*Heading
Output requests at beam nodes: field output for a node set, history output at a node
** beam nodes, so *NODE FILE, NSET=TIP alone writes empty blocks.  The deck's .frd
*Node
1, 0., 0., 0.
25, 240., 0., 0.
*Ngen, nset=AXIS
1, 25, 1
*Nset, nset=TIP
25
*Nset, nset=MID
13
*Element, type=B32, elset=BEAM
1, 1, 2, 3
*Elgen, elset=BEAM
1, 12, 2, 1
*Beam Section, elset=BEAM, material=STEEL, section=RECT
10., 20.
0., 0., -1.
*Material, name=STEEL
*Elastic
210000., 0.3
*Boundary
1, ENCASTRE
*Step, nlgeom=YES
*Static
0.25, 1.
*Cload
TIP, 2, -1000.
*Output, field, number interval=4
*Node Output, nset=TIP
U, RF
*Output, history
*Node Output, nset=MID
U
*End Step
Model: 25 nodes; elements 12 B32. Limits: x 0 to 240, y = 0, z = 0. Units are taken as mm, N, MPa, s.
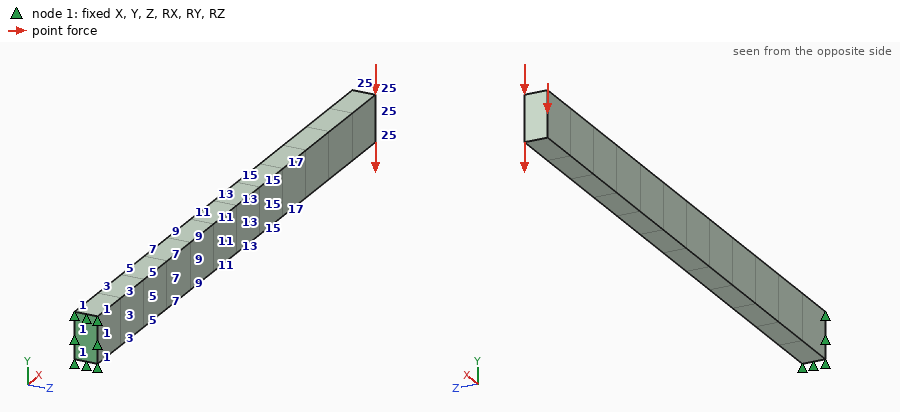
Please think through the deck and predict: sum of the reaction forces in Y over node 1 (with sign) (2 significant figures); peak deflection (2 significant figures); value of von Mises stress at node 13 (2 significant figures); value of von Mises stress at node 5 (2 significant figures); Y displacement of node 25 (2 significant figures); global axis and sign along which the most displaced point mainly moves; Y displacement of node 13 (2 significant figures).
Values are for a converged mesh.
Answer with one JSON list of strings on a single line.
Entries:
["1000 N", "3.3 mm", "180 MPa", "300 MPa", "-3.3 mm", "-Y", "-1.0 mm"]
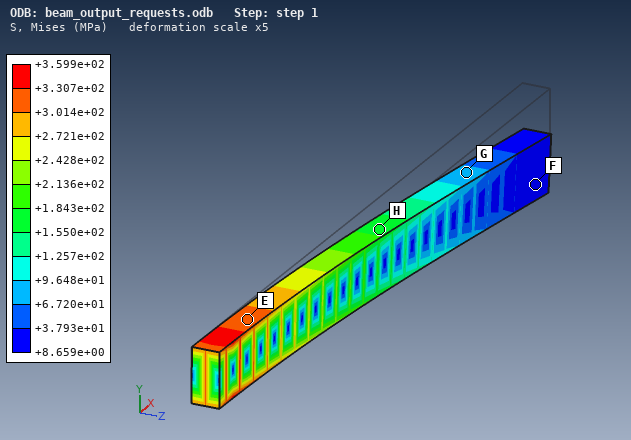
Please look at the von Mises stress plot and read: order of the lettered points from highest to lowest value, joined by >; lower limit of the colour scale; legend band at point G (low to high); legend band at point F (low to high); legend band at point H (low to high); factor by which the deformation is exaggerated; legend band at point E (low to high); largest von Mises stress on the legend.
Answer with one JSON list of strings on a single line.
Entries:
["E > H > G > F", "+8.659e+00 MPa", "+6.720e+01 to +9.648e+01 MPa", "+8.659e+00 to +3.793e+01 MPa", "+1.550e+02 to +1.843e+02 MPa", "5", "+3.014e+02 to +3.307e+02 MPa", "+3.599e+02 MPa"]
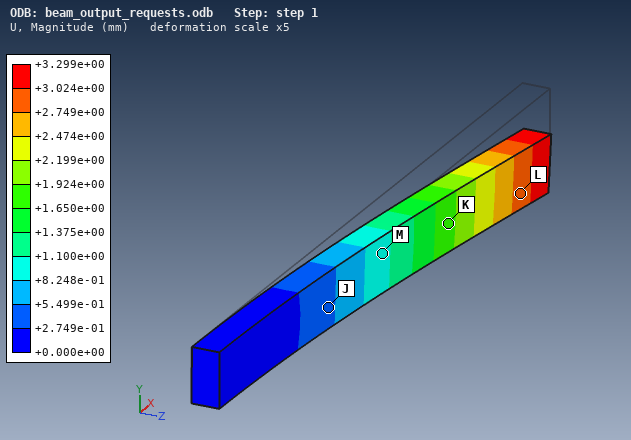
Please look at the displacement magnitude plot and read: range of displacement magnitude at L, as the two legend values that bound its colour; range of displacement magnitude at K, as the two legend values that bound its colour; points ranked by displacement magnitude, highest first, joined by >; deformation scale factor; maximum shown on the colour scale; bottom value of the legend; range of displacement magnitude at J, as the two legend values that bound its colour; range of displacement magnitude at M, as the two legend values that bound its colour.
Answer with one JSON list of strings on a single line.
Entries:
["+2.749e+00 to +3.024e+00 mm", "+1.650e+00 to +1.924e+00 mm", "L > K > M > J", "5", "+3.299e+00 mm", "+0.000e+00 mm", "+2.749e-01 to +5.499e-01 mm", "+8.248e-01 to +1.100e+00 mm"]
